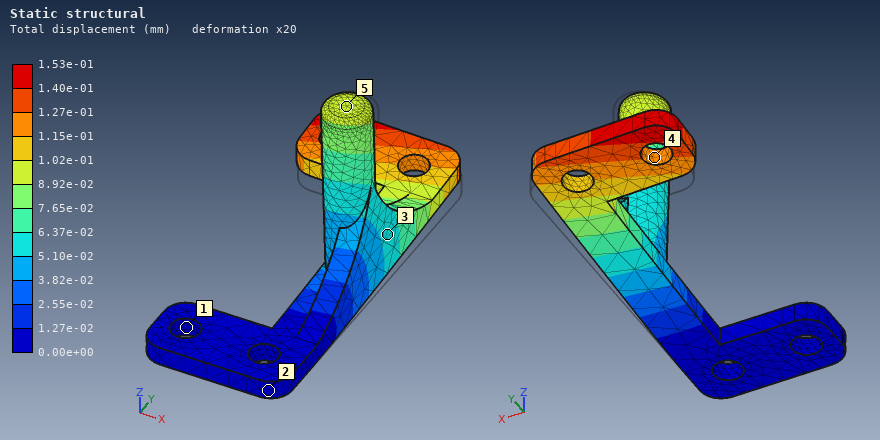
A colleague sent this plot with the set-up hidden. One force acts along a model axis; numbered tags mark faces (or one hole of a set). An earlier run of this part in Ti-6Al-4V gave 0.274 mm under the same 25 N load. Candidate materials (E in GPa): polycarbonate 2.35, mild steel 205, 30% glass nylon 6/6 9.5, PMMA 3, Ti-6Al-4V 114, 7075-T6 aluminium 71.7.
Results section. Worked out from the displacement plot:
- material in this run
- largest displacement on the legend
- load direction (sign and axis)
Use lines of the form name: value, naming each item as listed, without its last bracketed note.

material in this run: mild steel
largest displacement on the legend: 1.53e-01 mm
load direction: +Z
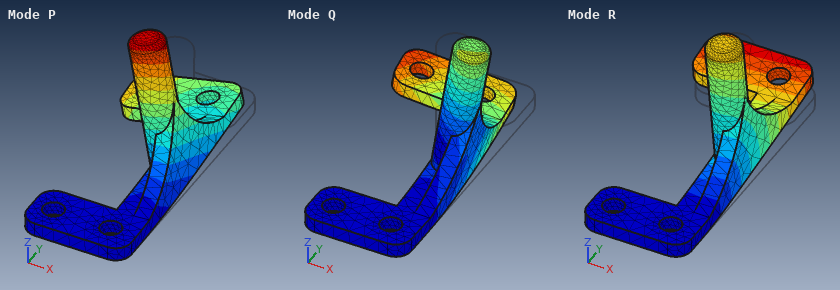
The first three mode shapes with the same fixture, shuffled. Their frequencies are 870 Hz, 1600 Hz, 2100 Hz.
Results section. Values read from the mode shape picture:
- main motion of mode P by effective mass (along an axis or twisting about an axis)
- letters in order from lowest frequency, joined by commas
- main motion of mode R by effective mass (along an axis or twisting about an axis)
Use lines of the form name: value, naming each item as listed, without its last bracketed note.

main motion of mode P by effective mass: along X
letters in order from lowest frequency, joined by commas: R, P, Q
main motion of mode R by effective mass: along Z
